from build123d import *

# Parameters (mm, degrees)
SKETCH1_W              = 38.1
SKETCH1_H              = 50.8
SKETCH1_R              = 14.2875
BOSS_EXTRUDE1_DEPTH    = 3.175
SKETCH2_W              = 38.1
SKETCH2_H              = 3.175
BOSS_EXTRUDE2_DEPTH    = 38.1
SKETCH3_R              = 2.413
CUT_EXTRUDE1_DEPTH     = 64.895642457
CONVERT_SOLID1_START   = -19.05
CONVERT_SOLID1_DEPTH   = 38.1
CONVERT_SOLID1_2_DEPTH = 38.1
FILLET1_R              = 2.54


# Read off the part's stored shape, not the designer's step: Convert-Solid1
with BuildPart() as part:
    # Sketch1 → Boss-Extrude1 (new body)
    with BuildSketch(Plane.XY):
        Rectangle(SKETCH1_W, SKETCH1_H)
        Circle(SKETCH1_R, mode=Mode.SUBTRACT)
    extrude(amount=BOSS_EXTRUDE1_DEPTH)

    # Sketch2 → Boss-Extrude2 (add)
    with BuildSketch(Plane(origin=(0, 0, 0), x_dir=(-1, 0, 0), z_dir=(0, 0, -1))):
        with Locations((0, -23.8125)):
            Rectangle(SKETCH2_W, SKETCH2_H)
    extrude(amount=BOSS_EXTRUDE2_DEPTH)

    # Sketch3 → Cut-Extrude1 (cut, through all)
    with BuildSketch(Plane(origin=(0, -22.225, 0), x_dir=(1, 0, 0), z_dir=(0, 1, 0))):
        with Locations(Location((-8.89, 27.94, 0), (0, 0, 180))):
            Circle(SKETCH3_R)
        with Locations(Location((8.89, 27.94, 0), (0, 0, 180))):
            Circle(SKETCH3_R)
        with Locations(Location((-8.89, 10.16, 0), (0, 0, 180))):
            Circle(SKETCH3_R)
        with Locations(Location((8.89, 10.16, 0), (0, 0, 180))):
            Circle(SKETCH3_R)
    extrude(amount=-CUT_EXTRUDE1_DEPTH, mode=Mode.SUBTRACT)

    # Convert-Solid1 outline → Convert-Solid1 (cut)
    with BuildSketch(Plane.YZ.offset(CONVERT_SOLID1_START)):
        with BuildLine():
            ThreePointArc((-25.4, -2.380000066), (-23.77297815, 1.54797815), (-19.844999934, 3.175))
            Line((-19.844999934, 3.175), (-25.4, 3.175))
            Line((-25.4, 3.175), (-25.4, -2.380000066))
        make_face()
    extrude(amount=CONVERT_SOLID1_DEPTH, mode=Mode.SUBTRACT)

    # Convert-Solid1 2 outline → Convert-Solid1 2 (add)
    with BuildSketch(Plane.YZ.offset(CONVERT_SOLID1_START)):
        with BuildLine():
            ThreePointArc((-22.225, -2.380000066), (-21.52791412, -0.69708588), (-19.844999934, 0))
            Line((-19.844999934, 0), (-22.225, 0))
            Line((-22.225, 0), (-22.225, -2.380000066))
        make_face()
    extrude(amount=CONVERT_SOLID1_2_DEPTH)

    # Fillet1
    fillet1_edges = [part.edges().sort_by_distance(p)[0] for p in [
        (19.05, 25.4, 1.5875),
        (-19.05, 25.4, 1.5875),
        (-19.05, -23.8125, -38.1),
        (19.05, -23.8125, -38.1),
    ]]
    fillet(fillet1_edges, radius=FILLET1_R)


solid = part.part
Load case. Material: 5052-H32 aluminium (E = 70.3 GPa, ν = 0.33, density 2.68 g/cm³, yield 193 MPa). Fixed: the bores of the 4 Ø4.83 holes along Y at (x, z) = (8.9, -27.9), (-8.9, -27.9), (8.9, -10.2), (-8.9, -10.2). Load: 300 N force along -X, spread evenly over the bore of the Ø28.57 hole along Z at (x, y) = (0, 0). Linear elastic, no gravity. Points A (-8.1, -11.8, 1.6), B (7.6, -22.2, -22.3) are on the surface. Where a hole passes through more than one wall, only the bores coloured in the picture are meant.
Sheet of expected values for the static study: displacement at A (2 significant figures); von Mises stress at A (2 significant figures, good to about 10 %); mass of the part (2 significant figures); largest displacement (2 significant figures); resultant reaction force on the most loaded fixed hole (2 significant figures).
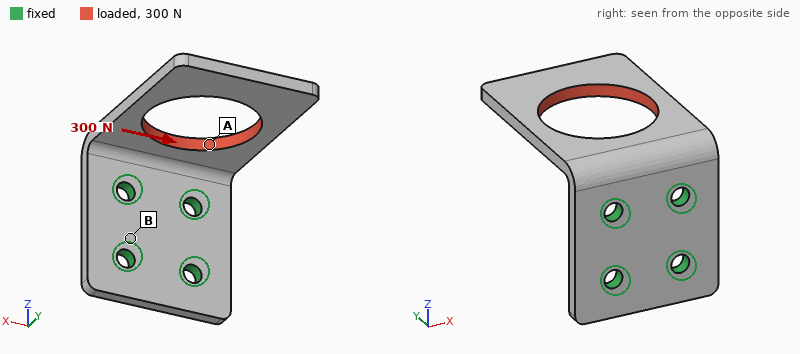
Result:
0.036 mm
29 MPa
22 g
0.15 mm
390 N
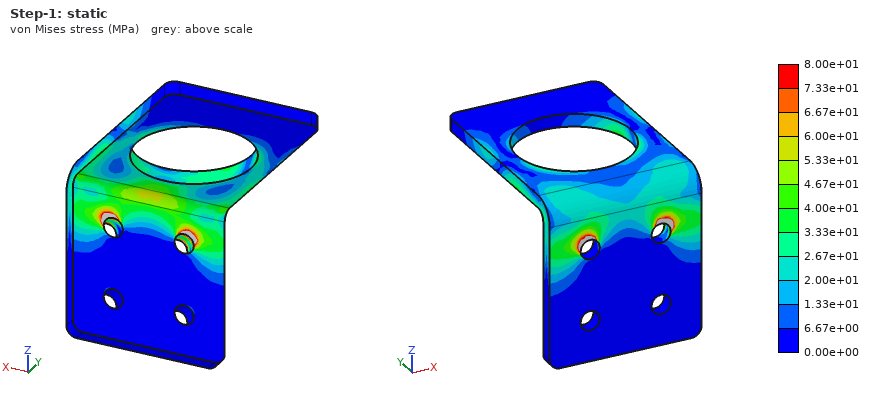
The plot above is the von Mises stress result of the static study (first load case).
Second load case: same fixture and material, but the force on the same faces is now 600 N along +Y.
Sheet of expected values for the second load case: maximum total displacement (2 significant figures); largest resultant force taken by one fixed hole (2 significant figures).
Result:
0.25 mm
330 N
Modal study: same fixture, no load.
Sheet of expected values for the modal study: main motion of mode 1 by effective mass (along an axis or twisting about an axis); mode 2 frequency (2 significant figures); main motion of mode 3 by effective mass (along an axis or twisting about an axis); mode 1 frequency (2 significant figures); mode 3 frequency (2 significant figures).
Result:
along Z
2100 Hz
along X
750 Hz
2800 Hz
